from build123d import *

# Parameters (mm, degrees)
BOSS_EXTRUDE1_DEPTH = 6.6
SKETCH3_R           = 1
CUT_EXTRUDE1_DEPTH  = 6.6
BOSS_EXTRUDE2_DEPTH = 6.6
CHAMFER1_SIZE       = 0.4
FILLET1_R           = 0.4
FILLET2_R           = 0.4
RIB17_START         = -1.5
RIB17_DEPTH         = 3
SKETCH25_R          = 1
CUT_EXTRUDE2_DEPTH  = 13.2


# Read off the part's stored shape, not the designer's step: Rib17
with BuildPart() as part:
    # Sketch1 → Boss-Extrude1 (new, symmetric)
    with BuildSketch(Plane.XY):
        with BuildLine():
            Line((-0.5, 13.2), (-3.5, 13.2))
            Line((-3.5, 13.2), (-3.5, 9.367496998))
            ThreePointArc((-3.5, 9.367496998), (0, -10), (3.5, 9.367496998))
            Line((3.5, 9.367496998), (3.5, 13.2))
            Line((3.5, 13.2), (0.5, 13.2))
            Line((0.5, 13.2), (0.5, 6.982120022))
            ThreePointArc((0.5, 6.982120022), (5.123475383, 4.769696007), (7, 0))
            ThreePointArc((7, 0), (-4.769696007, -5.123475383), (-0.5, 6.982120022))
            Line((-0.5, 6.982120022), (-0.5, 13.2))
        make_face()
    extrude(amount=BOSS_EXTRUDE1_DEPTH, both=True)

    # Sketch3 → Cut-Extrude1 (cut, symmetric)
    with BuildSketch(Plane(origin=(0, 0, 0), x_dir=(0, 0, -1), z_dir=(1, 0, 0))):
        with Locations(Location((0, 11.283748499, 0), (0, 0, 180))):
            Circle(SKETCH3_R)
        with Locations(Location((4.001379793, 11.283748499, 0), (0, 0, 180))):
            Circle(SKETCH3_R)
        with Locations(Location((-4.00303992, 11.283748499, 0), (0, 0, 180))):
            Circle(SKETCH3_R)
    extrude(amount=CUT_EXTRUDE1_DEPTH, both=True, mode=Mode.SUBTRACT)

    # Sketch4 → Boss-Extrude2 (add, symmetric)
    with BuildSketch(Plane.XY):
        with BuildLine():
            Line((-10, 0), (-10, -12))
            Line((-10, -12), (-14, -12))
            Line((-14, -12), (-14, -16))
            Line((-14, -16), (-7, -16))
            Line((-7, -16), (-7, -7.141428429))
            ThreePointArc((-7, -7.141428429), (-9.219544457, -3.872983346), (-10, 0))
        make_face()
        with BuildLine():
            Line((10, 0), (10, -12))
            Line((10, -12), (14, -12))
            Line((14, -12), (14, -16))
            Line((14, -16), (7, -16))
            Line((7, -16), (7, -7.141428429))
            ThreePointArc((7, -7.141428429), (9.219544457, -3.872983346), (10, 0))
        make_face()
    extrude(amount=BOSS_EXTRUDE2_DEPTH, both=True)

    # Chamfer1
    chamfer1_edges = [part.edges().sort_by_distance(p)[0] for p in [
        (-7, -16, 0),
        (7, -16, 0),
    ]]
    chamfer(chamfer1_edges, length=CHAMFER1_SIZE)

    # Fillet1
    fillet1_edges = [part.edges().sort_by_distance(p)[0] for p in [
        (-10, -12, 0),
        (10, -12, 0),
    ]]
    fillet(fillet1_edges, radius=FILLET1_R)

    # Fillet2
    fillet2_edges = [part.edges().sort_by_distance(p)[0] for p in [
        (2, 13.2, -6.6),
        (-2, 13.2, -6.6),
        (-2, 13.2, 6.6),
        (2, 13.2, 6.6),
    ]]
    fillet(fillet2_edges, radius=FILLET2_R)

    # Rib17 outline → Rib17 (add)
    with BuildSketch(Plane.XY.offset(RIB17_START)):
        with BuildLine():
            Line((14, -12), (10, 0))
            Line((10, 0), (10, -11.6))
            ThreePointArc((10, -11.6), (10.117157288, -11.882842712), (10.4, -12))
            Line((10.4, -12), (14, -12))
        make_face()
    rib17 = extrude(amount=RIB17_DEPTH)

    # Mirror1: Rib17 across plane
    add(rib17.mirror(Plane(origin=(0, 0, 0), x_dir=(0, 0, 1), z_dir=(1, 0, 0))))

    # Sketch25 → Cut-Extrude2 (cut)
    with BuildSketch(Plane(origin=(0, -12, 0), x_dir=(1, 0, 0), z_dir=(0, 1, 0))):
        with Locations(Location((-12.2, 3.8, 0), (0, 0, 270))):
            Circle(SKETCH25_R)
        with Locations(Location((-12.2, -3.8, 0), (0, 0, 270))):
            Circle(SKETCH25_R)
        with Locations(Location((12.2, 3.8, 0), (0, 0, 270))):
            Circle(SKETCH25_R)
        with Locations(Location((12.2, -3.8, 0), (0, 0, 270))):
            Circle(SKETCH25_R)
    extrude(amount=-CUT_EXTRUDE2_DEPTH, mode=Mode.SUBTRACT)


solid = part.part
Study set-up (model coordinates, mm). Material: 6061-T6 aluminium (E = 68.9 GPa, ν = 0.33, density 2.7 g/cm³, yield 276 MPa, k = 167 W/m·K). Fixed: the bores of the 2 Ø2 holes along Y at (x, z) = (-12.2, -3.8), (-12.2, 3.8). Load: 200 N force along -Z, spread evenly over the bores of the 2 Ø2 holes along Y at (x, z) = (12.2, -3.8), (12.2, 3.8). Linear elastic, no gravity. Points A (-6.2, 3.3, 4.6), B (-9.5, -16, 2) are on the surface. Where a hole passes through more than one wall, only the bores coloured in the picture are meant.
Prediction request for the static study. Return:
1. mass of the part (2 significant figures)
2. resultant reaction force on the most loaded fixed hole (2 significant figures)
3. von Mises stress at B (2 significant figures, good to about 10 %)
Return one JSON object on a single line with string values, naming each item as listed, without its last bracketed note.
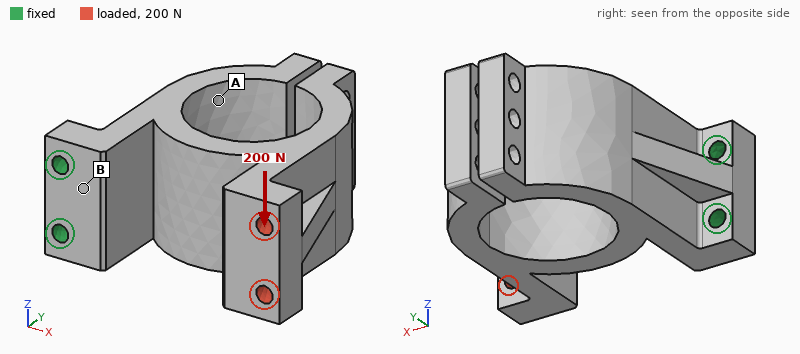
{"mass of the part": "9.9 g", "resultant reaction force on the most loaded fixed hole": "550 N", "von Mises stress at B": "46 MPa"}
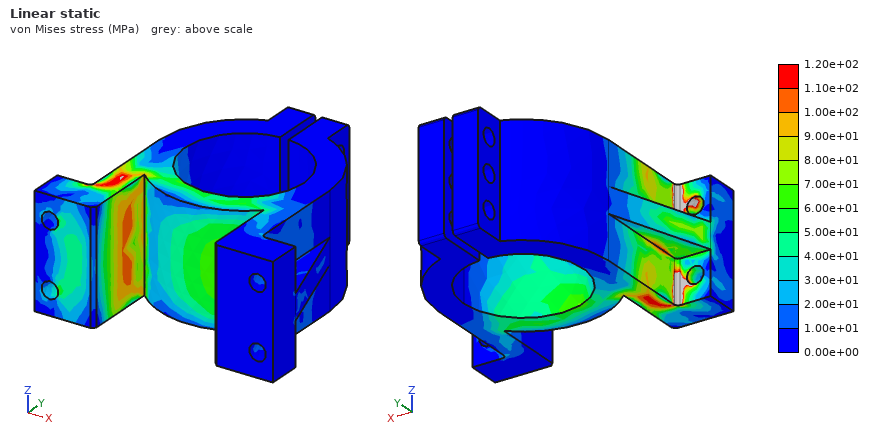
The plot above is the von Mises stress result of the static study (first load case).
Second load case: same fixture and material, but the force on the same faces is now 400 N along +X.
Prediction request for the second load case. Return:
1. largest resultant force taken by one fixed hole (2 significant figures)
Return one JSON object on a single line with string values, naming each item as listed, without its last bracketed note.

{"largest resultant force taken by one fixed hole": "200 N"}
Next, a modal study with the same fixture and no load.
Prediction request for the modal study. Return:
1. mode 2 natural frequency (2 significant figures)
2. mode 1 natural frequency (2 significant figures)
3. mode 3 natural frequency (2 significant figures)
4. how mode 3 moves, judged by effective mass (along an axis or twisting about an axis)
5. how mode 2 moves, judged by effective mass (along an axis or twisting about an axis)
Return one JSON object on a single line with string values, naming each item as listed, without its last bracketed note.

{"mode 2 natural frequency": "3100 Hz", "mode 1 natural frequency": "1600 Hz", "mode 3 natural frequency": "4200 Hz", "how mode 3 moves, judged by effective mass": "along Z", "how mode 2 moves, judged by effective mass": "along Z"}
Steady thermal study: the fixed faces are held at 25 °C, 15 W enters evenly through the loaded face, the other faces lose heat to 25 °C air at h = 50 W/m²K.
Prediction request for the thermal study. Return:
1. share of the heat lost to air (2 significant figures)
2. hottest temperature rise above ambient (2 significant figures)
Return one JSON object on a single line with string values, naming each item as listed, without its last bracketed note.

{"share of the heat lost to air": "27 %", "hottest temperature rise above ambient": "59 K"}
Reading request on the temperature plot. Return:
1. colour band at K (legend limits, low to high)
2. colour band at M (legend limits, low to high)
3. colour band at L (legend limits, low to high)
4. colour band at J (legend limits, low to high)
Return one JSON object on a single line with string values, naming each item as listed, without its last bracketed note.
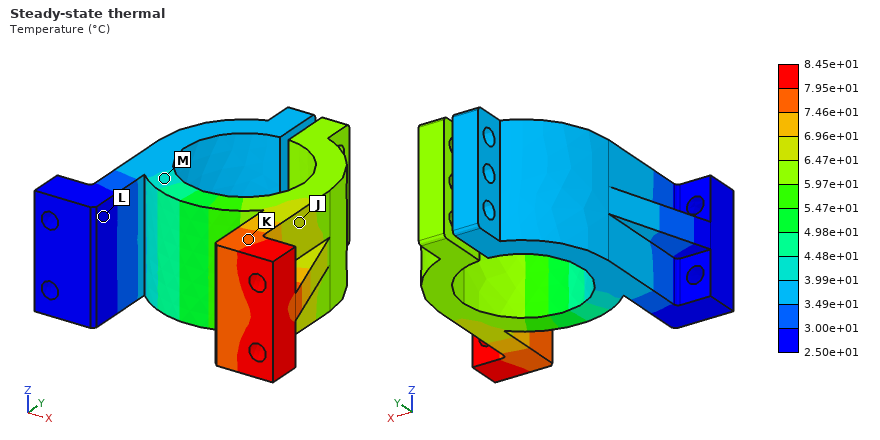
{"colour band at K": "7.46e+01 to 7.95e+01 °C", "colour band at M": "3.99e+01 to 4.48e+01 °C", "colour band at L": "2.50e+01 to 3.00e+01 °C", "colour band at J": "6.47e+01 to 6.96e+01 °C"}
